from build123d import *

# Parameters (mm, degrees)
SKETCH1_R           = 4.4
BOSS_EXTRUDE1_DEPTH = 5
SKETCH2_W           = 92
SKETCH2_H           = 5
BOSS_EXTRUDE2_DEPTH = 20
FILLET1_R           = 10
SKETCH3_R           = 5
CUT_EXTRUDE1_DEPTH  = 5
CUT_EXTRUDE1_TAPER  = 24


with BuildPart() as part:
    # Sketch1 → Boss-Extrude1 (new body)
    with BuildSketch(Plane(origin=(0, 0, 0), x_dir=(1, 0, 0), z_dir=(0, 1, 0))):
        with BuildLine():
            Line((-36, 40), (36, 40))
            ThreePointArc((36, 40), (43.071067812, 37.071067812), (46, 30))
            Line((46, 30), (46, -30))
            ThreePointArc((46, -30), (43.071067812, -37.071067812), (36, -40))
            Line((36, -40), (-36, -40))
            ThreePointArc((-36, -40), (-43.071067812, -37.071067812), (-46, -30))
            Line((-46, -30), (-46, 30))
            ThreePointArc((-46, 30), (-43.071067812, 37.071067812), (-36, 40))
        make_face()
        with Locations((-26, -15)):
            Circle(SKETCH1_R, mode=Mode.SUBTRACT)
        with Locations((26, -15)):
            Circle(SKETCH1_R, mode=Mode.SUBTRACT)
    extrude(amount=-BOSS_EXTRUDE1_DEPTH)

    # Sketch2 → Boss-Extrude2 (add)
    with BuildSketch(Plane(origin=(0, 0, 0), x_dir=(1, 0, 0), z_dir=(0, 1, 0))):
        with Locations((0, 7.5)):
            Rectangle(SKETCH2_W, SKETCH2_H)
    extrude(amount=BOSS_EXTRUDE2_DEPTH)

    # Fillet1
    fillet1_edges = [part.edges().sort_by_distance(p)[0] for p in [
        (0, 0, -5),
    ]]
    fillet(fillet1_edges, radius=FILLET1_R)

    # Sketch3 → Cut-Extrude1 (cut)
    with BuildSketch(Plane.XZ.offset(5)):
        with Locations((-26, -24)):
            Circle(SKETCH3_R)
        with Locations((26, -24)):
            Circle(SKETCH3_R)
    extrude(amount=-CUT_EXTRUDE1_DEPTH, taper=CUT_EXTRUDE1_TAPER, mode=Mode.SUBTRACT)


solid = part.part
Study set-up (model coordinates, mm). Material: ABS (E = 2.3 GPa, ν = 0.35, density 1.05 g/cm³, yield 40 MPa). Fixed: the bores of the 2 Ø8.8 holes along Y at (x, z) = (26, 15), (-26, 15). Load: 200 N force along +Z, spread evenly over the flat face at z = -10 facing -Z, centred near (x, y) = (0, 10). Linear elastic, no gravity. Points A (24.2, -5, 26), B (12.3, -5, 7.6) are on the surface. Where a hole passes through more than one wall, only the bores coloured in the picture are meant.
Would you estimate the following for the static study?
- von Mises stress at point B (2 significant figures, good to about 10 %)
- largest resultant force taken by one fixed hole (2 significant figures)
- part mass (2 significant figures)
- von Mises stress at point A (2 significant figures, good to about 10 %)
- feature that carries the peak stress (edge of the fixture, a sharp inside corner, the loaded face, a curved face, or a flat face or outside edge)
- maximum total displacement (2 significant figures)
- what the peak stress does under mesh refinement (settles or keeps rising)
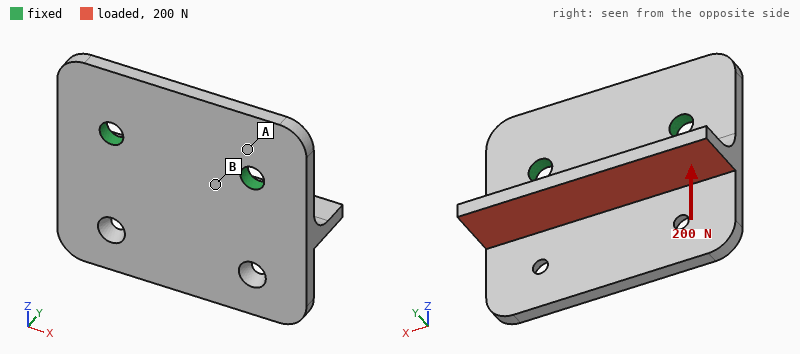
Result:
4.5 MPa
100 N
49 g
1.3 MPa
edge of the fixture
0.75 mm
keeps rising
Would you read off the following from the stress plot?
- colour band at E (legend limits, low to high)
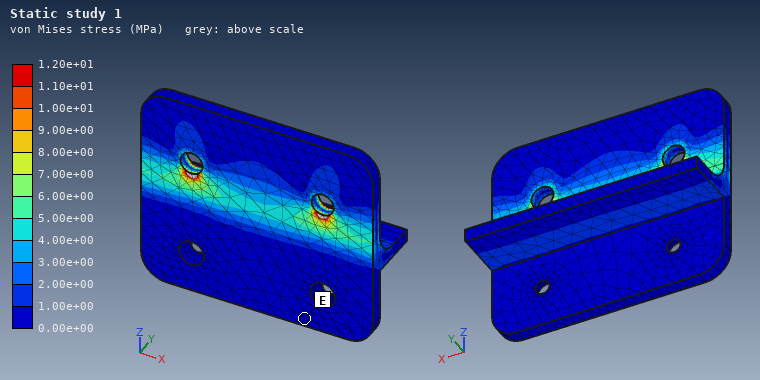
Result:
0.00e+00 to 1.00e+00 MPa
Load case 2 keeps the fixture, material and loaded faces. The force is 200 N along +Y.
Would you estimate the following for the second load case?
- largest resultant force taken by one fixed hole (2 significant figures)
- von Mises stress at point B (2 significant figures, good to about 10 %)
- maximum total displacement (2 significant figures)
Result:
100 N
6.1 MPa
1.1 mm
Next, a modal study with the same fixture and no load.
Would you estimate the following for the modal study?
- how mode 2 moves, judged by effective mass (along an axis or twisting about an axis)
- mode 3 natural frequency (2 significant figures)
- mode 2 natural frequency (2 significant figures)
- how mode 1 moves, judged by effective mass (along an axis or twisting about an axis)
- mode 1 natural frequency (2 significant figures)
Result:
twisting about Z
1800 Hz
770 Hz
along Y
420 Hz
